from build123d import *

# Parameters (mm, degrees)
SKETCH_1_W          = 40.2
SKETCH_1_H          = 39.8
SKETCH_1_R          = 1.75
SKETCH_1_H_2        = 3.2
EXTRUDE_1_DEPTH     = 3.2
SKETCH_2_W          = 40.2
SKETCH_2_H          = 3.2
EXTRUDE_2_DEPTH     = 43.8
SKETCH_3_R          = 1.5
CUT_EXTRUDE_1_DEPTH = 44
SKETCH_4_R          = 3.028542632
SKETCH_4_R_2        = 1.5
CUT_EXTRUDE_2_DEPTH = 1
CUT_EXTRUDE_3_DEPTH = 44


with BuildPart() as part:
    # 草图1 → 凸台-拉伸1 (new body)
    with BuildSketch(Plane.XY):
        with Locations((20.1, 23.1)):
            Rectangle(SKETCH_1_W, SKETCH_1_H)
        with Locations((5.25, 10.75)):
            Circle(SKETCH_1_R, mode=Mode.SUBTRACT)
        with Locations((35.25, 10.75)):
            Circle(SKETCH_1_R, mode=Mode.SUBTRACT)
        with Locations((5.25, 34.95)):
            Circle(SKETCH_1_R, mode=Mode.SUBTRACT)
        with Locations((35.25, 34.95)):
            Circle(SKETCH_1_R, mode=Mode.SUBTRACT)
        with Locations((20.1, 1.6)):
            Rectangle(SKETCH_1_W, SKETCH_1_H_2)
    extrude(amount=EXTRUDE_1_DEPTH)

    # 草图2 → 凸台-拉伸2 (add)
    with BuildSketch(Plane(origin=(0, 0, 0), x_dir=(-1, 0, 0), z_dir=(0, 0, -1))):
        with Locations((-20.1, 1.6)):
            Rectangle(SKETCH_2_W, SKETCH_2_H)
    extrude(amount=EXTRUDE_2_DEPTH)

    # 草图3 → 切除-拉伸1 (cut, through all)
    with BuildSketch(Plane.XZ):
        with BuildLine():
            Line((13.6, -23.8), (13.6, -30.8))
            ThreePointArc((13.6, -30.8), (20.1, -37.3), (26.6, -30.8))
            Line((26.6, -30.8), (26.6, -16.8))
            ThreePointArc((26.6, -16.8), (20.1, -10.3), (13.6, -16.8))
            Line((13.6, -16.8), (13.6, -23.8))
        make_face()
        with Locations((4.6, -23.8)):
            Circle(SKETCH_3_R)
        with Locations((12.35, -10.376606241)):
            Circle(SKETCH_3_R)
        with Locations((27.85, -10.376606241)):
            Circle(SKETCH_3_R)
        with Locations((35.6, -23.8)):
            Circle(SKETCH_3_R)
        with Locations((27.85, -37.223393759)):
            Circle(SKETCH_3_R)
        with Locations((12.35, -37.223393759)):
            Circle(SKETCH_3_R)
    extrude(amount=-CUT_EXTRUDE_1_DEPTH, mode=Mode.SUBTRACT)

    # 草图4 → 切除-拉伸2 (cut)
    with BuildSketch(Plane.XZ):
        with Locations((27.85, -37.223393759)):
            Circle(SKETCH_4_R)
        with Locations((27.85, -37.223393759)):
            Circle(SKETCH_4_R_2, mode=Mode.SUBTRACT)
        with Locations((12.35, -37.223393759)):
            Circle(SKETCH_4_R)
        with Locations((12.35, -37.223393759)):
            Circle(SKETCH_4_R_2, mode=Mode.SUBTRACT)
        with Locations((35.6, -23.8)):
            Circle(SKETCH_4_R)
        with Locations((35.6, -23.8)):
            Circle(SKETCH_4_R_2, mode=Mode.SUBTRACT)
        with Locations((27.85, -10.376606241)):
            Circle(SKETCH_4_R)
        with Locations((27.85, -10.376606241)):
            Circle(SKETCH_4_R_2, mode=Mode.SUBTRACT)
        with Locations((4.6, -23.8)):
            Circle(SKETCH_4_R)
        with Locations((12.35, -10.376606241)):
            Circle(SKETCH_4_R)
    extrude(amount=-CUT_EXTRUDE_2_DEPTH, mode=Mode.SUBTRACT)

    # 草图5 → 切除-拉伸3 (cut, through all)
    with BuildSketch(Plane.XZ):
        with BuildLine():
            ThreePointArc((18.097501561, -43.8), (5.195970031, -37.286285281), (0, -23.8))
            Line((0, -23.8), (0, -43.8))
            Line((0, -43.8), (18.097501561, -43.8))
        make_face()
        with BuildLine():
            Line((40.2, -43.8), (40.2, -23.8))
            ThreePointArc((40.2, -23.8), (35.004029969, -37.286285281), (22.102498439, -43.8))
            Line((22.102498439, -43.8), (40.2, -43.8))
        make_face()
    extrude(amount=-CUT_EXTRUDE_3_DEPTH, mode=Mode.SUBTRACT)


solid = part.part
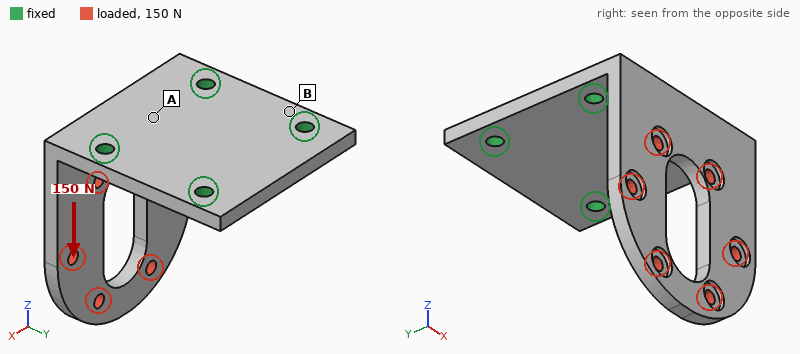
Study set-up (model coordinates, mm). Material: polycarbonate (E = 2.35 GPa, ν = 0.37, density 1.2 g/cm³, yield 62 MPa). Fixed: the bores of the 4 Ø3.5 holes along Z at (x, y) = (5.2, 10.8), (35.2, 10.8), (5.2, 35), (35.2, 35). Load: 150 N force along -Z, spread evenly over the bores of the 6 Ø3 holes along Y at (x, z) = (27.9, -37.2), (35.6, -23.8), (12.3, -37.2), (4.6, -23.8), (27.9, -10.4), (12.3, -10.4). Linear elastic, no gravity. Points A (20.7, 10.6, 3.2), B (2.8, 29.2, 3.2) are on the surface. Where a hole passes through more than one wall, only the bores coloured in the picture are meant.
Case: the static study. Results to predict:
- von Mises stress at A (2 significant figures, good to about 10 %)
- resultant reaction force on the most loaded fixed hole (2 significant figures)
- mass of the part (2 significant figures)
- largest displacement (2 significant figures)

4.6 MPa
81 N
11 g
0.78 mm
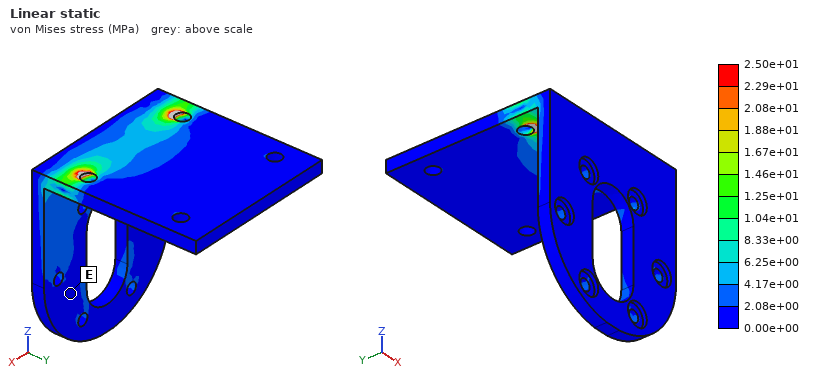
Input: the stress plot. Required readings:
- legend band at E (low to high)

0.00e+00 to 2.08e+00 MPa
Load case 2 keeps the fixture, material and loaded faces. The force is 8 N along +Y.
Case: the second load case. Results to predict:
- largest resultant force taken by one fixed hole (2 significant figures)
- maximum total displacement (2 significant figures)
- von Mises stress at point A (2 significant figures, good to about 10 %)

3.2 N
0.79 mm
1.4 MPa
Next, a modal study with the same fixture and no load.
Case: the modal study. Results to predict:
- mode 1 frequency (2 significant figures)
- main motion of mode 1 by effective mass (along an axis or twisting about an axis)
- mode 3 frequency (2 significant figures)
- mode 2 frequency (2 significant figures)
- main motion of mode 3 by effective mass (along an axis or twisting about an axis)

350 Hz
along Y
1400 Hz
880 Hz
along X
